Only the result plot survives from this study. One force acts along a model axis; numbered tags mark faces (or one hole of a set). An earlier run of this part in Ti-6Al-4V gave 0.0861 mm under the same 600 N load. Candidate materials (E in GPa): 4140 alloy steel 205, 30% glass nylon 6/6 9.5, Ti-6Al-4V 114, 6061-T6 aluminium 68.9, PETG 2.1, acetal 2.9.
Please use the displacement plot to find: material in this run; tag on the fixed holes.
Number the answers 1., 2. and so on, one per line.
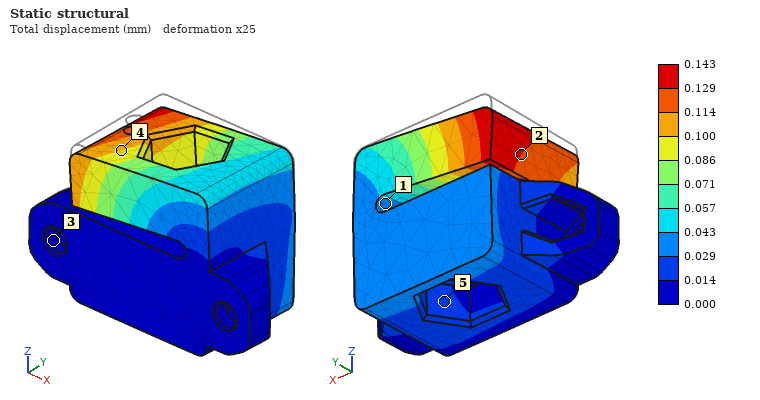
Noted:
1. 6061-T6 aluminium
2. 3
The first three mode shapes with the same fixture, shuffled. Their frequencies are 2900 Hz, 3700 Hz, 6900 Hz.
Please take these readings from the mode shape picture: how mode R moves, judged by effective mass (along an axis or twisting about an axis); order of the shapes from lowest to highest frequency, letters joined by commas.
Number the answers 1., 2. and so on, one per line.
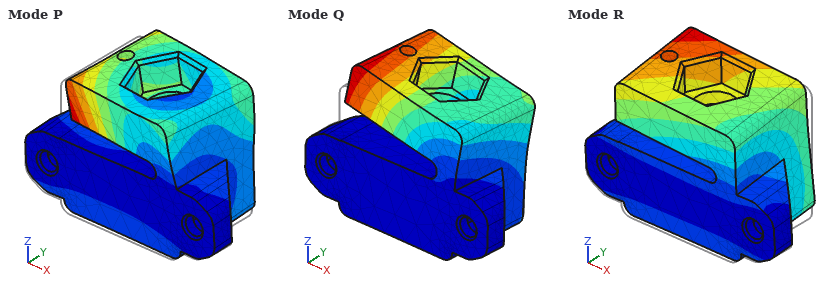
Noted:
1. along Z
2. R, Q, P
